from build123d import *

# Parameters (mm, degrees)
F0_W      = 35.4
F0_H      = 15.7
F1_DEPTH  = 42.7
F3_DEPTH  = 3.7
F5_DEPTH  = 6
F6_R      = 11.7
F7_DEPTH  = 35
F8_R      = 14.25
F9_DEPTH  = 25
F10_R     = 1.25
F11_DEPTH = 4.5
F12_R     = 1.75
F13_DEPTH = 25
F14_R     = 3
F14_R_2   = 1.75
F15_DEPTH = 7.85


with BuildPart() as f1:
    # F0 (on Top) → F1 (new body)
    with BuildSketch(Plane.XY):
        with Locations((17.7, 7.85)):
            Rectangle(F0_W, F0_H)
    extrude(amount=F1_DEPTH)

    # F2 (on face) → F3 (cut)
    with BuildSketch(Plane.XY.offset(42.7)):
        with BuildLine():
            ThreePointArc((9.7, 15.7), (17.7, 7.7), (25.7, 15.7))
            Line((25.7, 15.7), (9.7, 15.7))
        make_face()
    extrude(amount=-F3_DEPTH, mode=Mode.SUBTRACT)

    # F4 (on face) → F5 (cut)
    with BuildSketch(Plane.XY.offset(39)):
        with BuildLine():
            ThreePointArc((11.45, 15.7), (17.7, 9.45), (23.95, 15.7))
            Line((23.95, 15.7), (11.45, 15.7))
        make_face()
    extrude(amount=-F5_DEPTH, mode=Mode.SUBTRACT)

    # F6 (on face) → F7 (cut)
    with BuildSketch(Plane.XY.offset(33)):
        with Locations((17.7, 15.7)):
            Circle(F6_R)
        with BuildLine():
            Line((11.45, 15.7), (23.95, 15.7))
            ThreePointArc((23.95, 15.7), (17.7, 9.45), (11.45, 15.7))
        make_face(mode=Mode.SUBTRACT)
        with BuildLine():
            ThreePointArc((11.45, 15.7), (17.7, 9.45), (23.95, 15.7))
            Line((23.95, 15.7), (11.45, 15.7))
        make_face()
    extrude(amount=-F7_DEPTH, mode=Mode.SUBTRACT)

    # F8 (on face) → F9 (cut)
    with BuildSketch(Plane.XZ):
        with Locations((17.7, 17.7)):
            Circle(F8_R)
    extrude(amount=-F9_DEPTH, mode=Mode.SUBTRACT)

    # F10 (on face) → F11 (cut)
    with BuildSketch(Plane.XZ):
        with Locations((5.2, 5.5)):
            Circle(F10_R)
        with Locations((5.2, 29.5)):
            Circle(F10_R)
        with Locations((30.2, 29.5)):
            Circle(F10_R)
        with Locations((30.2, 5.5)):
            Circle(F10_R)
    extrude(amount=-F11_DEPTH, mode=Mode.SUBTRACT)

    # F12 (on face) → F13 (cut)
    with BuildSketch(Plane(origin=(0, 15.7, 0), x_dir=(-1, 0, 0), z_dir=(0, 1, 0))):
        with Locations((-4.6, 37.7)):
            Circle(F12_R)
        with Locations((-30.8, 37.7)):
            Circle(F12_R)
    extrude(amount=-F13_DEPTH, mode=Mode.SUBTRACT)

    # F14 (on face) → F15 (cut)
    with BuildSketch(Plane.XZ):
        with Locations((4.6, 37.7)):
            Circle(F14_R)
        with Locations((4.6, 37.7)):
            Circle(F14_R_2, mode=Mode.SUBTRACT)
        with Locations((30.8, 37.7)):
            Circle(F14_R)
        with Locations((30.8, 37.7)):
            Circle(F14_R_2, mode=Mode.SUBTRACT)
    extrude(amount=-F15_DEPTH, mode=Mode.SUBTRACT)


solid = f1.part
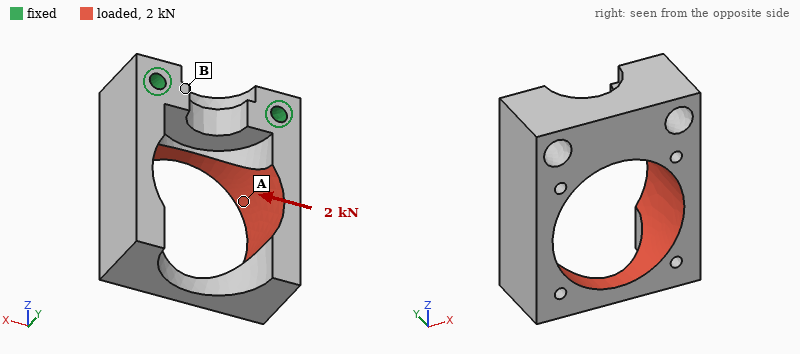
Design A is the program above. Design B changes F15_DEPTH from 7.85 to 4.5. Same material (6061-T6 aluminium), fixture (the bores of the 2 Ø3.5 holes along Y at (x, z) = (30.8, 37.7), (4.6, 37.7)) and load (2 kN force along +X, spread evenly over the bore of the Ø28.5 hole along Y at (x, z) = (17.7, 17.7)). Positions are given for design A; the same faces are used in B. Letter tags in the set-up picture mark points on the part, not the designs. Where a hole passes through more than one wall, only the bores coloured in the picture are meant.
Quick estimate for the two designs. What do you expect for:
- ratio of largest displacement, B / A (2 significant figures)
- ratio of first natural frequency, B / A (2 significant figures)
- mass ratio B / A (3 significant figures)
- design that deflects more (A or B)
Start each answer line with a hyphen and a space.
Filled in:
- 0.87
- 1.1
- 1.01
- A
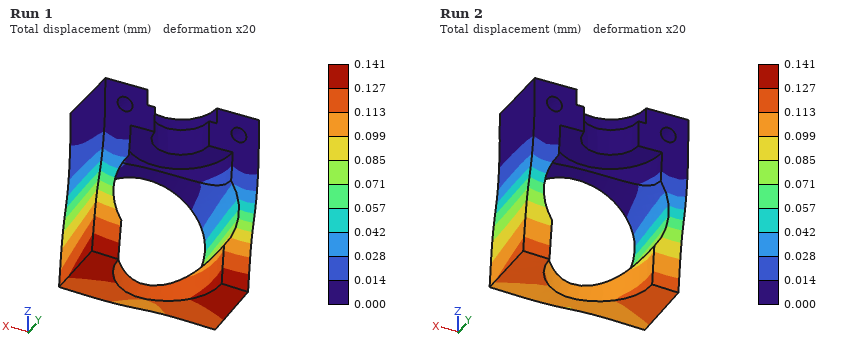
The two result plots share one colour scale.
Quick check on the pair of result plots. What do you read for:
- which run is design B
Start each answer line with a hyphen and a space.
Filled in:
- Run 2
